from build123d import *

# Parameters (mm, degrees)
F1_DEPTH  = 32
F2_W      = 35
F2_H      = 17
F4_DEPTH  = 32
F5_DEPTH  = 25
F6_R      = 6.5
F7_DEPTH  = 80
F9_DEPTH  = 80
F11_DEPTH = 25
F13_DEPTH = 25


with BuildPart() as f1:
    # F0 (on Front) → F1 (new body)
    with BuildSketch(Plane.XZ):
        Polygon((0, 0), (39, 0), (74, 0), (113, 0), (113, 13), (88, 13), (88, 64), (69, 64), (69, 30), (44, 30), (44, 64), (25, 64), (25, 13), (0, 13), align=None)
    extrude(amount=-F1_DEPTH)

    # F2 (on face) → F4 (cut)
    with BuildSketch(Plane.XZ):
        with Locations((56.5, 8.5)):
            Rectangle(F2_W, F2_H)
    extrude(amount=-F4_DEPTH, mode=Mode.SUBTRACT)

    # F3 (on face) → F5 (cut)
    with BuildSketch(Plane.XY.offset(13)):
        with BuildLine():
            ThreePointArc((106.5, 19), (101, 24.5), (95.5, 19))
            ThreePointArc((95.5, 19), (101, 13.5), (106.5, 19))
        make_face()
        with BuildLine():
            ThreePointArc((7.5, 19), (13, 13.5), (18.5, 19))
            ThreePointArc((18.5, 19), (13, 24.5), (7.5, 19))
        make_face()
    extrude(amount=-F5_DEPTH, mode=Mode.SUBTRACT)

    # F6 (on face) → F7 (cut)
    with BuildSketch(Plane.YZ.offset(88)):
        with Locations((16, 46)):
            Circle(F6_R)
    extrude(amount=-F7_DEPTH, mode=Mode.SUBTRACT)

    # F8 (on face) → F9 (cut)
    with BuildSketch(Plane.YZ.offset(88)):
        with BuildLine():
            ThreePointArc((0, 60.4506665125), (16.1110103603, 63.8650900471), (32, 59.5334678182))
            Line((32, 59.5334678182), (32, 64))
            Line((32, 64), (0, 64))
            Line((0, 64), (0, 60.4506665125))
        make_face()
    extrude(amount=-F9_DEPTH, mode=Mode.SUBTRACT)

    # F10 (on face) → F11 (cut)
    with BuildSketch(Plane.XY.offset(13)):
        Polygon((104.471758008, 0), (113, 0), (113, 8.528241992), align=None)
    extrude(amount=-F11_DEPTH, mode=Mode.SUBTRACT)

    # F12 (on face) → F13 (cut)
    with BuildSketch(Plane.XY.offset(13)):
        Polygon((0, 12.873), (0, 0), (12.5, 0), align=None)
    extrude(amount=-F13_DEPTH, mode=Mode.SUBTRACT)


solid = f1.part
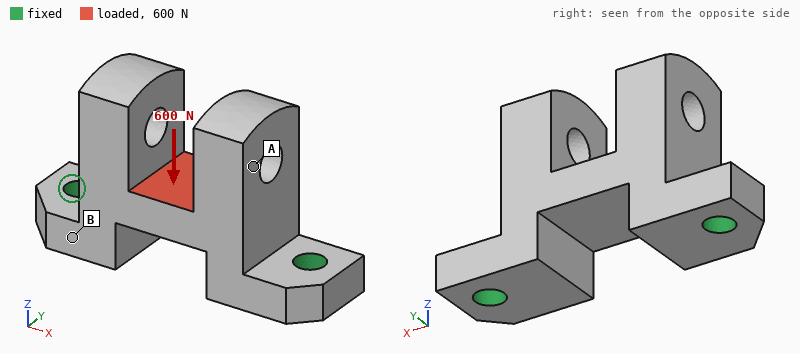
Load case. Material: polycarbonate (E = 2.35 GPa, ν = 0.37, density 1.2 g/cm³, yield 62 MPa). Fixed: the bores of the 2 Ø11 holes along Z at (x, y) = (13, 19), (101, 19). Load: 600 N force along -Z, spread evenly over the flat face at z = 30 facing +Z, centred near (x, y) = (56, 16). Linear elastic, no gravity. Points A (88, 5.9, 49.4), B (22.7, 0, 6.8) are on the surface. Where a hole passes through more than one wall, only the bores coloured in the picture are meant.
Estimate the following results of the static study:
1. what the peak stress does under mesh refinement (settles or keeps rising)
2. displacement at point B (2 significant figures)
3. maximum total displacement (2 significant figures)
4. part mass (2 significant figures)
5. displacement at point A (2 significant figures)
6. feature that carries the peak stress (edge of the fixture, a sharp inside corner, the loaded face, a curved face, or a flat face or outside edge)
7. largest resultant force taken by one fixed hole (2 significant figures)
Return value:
keeps rising
24 µm
92 µm
110 g
56 µm
edge of the fixture
450 N
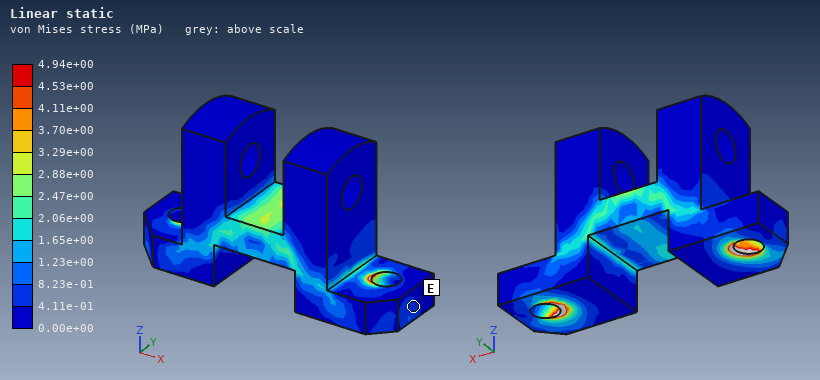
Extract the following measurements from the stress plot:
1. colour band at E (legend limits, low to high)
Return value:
4.11e-01 to 8.23e-01 MPa
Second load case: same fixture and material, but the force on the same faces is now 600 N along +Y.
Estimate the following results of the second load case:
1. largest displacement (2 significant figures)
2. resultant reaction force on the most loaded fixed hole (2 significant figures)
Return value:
0.40 mm
300 N
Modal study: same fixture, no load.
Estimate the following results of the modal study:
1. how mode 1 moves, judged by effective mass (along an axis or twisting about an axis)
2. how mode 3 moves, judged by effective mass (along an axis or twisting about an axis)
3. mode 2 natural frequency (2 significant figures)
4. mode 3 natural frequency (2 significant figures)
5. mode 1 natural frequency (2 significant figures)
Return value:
along Y
along X
1300 Hz
1600 Hz
760 Hz
